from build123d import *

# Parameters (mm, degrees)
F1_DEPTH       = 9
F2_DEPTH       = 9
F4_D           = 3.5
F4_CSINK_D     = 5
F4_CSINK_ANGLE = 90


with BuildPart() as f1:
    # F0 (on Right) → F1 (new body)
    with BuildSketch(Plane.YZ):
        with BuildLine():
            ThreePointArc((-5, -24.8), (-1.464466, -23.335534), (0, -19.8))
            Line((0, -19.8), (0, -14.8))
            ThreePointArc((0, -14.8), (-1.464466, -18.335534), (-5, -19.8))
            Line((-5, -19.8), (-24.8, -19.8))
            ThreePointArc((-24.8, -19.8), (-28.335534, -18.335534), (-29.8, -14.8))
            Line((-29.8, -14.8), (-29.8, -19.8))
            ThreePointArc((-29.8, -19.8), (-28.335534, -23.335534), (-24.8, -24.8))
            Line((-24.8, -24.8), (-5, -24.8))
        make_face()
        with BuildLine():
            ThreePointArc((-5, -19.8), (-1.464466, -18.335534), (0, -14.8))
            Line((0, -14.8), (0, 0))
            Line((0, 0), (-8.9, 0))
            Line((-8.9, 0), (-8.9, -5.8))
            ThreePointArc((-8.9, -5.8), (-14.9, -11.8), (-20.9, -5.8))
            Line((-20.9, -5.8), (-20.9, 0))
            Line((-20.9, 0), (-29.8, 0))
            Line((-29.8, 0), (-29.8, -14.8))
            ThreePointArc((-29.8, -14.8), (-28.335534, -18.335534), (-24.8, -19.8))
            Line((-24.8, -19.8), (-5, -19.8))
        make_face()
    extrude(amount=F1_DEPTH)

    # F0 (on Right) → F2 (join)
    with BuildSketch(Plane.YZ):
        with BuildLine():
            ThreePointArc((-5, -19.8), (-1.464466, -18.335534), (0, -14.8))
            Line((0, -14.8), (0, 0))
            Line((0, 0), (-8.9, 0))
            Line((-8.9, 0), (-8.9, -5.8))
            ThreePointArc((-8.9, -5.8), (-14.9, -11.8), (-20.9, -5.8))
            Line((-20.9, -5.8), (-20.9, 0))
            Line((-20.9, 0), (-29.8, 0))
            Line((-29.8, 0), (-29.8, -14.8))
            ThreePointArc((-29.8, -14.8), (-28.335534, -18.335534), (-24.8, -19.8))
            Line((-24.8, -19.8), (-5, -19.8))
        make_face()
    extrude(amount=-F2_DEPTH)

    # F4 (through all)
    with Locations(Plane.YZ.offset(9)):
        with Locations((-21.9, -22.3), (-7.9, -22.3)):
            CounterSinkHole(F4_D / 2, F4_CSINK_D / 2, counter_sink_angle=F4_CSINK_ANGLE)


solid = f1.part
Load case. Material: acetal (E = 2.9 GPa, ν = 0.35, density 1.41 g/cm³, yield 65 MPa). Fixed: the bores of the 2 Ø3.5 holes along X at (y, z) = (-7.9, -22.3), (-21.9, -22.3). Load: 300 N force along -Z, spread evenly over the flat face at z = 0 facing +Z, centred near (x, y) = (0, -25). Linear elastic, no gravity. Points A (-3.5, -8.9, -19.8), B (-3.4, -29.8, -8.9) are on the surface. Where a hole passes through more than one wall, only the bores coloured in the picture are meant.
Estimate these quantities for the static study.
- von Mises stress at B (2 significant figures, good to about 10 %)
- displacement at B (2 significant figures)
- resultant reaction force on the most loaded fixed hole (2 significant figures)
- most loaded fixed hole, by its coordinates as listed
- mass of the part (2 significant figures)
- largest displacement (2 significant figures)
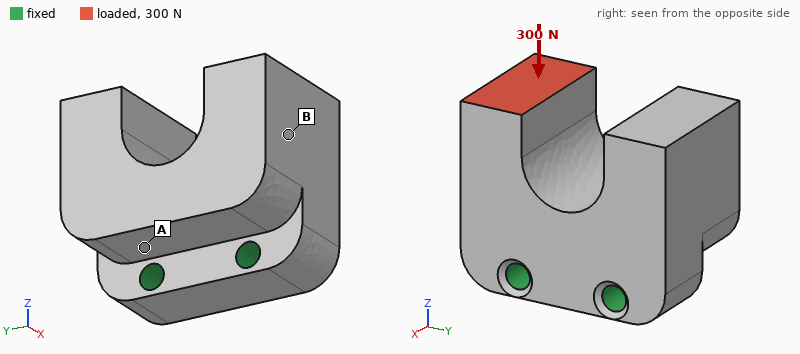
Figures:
2.3 MPa
0.064 mm
340 N
(-21.9, -22.3)
13 g
0.10 mm
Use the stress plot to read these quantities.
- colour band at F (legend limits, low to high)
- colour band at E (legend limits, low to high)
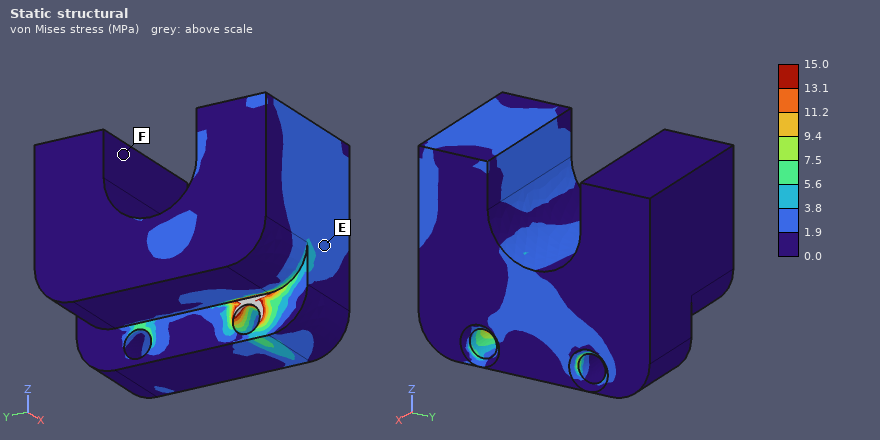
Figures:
0.0 to 1.9 MPa
1.9 to 3.8 MPa
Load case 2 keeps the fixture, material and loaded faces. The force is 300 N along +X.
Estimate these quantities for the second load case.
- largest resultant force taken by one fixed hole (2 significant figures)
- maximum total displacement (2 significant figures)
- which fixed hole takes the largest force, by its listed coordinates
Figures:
280 N
0.41 mm
(-21.9, -22.3)
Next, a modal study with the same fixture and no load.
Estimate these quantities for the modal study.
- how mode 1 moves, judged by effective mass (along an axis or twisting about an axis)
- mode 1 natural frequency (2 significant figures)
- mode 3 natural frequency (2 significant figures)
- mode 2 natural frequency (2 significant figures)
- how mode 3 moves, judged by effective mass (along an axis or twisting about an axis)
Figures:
along X
2700 Hz
4600 Hz
4100 Hz
along Y
